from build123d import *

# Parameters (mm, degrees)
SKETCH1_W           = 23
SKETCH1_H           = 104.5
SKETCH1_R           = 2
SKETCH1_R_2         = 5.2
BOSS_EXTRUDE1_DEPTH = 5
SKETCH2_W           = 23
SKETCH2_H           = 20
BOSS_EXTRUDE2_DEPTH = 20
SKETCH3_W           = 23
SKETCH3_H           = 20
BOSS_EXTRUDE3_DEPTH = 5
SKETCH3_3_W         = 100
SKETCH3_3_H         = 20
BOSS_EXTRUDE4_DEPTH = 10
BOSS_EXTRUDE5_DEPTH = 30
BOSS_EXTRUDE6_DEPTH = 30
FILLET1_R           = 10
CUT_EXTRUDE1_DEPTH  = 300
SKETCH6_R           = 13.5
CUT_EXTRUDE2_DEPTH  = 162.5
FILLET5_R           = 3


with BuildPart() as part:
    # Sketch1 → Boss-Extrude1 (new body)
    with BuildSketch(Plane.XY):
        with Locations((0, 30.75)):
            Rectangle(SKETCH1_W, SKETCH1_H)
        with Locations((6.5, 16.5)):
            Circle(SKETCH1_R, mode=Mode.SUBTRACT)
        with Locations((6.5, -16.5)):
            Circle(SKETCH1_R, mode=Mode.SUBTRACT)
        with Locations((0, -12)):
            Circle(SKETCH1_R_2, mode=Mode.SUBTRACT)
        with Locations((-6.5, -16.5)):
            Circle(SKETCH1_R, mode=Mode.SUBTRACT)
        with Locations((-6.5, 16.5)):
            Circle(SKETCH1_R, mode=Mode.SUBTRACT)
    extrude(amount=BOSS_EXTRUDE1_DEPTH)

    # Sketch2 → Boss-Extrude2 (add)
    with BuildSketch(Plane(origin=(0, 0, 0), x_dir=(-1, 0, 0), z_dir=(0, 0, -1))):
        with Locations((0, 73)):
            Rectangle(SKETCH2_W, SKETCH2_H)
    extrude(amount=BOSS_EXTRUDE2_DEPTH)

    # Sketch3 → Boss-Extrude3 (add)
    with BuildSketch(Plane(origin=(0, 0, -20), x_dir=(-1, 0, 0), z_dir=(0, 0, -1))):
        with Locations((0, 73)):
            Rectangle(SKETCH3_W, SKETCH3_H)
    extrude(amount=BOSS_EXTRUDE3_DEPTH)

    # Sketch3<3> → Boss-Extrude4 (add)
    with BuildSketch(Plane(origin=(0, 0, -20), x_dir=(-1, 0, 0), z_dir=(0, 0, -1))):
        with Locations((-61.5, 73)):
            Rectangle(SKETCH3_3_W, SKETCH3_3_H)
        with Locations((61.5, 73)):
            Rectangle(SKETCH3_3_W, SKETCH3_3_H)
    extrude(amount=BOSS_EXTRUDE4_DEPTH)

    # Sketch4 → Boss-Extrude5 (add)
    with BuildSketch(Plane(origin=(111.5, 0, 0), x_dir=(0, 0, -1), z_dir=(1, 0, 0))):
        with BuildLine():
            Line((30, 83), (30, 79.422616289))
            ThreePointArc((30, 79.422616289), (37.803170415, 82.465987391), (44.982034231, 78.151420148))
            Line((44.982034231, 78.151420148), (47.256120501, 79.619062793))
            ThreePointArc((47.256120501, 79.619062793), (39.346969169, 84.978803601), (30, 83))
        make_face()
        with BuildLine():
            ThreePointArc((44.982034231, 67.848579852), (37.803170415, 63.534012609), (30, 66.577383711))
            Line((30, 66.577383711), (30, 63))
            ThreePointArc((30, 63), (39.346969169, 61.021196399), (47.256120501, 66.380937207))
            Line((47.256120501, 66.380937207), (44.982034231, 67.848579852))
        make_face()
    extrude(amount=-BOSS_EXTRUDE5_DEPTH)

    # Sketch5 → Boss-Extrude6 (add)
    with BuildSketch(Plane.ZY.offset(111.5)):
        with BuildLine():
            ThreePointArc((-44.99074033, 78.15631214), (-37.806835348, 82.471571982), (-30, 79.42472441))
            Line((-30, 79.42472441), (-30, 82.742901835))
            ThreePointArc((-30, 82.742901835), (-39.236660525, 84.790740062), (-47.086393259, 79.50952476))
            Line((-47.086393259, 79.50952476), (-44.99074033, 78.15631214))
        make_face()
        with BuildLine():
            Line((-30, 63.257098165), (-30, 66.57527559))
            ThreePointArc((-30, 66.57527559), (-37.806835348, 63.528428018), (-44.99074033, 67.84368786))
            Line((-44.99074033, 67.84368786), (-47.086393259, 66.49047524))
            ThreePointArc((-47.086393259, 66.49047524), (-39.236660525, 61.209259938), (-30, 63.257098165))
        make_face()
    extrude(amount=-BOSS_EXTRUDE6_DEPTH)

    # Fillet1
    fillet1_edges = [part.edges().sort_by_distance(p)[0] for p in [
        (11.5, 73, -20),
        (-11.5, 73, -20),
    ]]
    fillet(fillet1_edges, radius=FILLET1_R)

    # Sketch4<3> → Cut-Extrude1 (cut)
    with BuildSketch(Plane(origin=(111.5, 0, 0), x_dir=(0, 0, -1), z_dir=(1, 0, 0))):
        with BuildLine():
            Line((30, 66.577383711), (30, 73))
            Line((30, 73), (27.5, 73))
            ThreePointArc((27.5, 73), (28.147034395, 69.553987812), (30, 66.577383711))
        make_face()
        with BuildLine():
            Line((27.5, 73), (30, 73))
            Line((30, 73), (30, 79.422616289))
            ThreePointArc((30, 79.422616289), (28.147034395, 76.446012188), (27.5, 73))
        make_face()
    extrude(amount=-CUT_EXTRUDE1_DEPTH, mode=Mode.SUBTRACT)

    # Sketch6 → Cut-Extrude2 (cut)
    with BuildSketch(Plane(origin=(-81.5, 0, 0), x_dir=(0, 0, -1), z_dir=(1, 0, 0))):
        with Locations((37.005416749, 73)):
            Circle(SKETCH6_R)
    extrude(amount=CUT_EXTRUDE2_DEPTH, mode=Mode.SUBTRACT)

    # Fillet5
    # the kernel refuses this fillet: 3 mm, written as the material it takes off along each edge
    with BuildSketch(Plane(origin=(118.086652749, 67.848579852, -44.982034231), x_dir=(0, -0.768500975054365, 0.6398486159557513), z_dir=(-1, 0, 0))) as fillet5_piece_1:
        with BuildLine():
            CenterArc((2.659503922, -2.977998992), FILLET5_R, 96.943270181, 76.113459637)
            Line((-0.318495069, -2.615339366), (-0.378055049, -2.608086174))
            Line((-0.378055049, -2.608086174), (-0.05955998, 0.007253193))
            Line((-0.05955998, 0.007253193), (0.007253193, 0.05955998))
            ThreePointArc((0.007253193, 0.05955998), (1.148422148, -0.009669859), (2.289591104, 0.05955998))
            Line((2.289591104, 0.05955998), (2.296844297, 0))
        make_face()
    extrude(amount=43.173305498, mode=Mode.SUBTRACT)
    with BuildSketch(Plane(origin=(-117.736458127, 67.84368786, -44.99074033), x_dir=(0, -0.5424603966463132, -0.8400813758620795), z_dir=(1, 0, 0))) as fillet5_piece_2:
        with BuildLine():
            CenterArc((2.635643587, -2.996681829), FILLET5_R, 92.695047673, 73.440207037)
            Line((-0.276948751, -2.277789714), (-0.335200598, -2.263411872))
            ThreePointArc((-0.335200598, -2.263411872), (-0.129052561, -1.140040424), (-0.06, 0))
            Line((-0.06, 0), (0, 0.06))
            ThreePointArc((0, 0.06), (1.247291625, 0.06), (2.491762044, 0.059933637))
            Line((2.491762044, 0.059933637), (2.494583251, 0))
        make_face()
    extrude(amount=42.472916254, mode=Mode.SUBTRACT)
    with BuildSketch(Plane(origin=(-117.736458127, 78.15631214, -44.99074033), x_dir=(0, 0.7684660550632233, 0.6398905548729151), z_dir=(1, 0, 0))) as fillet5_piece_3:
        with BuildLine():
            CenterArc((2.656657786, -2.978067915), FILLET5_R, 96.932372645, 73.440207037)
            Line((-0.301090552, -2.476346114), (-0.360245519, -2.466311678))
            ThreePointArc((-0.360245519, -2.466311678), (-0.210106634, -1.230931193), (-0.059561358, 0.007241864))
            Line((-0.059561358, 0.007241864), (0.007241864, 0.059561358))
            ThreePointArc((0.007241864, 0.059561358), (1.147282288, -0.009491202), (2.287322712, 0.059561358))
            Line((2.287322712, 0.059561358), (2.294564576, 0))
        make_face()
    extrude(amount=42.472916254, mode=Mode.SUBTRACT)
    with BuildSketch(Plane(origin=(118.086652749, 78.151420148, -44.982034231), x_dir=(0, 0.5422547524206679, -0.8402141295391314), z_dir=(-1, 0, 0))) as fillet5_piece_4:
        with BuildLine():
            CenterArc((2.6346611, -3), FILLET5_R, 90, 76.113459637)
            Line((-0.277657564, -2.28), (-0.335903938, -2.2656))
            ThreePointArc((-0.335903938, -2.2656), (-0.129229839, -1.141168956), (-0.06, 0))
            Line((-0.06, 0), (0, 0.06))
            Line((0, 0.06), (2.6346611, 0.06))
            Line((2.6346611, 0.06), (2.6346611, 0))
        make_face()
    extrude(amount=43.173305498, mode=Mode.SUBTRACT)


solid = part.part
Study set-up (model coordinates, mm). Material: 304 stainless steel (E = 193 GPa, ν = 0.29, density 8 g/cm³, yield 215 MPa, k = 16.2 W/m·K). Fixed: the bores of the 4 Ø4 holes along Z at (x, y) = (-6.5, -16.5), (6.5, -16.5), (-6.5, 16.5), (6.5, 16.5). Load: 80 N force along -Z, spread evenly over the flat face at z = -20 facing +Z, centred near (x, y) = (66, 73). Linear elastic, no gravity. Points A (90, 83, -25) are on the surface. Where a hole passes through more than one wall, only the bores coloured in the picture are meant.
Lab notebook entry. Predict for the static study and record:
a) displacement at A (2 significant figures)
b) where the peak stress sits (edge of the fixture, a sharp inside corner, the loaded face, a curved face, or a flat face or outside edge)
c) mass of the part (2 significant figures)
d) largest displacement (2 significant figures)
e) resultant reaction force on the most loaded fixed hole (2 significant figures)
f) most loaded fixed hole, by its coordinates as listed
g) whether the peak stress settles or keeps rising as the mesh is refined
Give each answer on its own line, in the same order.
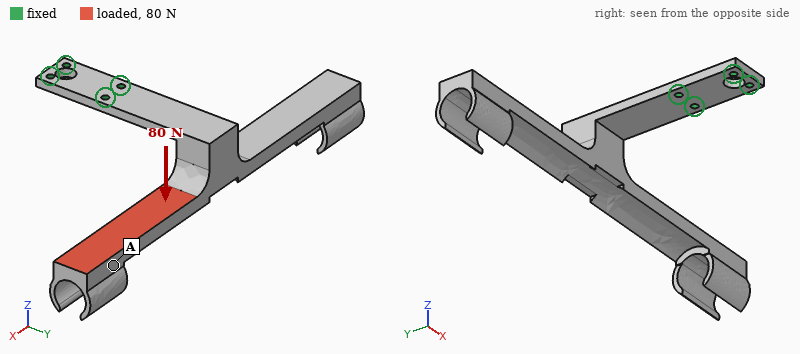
0.57 mm
edge of the fixture
430 g
0.72 mm
350 N
(6.5, 16.5)
keeps rising
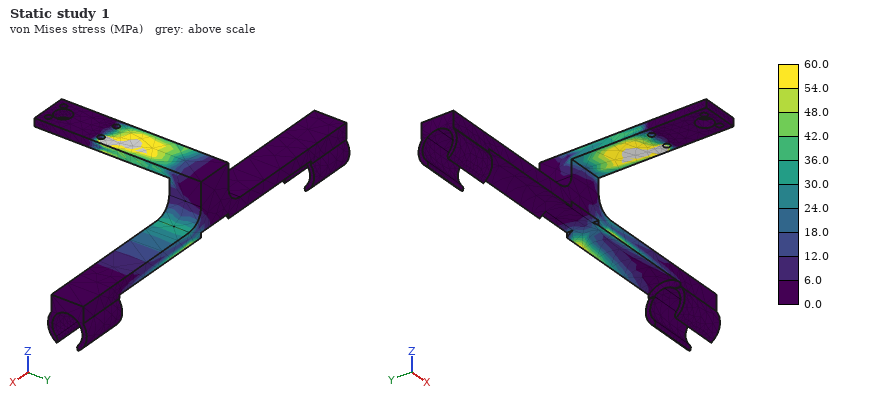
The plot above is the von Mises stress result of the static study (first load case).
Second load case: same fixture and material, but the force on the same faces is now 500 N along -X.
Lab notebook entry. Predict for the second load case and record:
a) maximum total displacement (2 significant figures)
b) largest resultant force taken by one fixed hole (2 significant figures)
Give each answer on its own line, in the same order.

0.86 mm
1.9 kN
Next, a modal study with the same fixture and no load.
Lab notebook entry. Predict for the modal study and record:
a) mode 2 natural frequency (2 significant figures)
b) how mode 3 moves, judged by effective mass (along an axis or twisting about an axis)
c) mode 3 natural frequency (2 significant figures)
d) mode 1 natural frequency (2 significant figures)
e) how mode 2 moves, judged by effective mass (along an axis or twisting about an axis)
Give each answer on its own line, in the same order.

180 Hz
along Y
380 Hz
140 Hz
along Z
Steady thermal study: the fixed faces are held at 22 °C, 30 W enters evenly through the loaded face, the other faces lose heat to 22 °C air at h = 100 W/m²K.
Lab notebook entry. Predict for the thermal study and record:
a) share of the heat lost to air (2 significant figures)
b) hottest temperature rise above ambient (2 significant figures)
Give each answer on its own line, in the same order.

100 %
74 K
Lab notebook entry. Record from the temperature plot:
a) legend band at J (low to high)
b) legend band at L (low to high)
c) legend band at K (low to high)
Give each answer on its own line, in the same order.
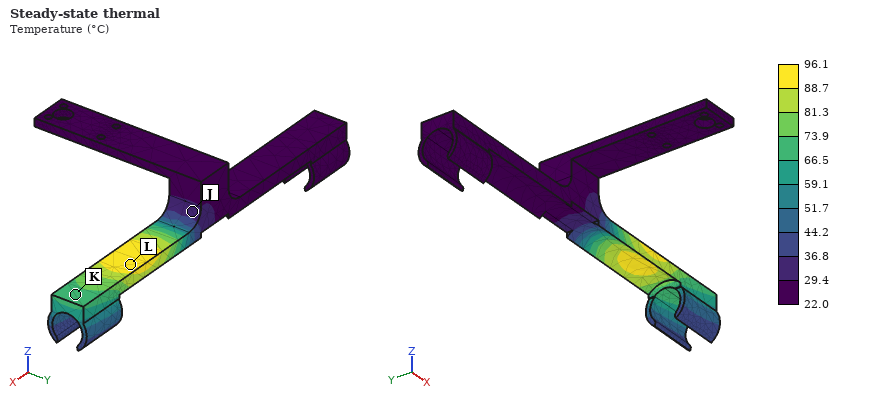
29.4 to 36.8 °C
88.7 to 96.1 °C
66.5 to 73.9 °C
